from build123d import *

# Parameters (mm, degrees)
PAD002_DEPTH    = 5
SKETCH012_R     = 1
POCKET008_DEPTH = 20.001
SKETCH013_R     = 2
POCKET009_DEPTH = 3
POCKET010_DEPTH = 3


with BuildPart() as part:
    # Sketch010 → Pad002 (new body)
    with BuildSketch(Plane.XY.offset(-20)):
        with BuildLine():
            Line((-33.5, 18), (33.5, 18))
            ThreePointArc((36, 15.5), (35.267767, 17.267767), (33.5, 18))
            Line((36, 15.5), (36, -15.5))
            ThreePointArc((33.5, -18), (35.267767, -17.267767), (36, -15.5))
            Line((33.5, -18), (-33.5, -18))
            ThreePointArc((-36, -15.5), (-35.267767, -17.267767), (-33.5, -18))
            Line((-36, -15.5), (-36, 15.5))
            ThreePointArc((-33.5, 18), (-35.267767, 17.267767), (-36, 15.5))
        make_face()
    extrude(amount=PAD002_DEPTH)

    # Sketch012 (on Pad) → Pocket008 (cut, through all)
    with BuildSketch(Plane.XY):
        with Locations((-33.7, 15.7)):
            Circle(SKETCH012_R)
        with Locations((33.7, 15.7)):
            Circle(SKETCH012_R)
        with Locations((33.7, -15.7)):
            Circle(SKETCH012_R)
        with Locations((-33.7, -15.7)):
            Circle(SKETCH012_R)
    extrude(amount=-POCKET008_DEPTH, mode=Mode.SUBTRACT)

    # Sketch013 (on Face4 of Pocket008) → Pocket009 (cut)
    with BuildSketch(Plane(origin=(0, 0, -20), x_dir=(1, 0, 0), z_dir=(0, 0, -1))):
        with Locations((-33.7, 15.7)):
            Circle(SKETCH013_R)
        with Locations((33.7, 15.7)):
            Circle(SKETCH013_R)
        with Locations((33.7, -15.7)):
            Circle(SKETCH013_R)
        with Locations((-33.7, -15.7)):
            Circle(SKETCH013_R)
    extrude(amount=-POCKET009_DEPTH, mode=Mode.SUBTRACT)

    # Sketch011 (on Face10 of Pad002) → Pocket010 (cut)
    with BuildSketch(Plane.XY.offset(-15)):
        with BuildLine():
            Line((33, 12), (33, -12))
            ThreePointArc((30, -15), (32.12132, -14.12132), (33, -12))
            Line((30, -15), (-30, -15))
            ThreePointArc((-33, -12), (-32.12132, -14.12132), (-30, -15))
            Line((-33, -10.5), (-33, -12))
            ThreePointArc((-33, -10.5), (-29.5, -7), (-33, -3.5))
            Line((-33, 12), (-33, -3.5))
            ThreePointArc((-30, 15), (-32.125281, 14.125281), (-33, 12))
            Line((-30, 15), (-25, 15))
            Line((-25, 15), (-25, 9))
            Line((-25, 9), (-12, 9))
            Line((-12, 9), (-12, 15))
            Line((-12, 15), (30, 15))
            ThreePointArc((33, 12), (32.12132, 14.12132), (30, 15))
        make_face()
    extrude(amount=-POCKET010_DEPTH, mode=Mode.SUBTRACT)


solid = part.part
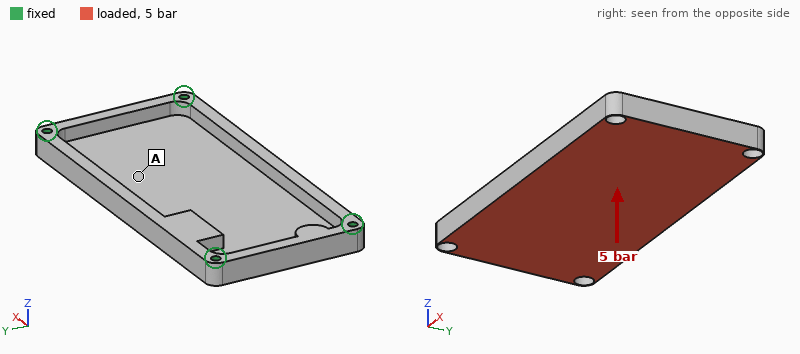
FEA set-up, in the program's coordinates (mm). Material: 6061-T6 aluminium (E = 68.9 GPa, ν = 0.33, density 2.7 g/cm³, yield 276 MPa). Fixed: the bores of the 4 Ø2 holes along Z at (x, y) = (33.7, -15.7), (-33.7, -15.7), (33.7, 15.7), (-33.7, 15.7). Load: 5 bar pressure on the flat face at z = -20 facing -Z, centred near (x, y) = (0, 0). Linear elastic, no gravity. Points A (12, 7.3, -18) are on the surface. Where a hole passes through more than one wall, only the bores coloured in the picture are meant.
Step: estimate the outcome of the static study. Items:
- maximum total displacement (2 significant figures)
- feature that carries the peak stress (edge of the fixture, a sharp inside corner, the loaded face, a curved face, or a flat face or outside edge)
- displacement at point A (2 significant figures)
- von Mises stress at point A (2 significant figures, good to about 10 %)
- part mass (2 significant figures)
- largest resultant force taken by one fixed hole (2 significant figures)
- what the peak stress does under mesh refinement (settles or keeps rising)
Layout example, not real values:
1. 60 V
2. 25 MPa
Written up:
1. 0.23 mm
2. edge of the fixture
3. 0.18 mm
4. 32 MPa
5. 19 g
6. 790 N
7. keeps rising
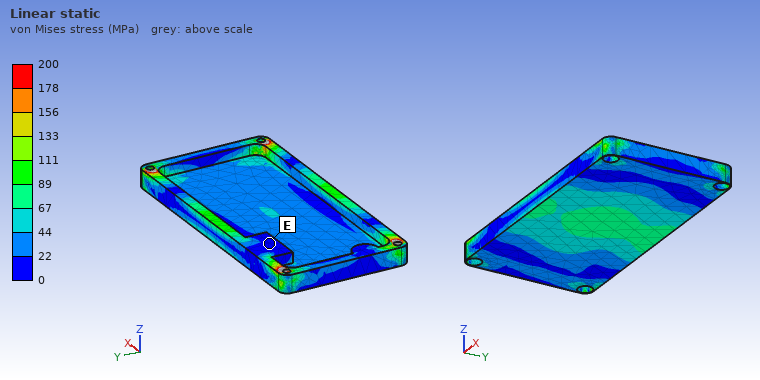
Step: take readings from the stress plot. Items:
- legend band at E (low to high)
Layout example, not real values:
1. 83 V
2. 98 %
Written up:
1. 0 to 22 MPa
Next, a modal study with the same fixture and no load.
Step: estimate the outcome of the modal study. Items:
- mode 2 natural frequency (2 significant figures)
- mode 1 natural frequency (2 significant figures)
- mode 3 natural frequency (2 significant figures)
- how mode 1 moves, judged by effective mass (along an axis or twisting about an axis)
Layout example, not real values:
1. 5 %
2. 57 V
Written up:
1. 4900 Hz
2. 3500 Hz
3. 7900 Hz
4. along Z
